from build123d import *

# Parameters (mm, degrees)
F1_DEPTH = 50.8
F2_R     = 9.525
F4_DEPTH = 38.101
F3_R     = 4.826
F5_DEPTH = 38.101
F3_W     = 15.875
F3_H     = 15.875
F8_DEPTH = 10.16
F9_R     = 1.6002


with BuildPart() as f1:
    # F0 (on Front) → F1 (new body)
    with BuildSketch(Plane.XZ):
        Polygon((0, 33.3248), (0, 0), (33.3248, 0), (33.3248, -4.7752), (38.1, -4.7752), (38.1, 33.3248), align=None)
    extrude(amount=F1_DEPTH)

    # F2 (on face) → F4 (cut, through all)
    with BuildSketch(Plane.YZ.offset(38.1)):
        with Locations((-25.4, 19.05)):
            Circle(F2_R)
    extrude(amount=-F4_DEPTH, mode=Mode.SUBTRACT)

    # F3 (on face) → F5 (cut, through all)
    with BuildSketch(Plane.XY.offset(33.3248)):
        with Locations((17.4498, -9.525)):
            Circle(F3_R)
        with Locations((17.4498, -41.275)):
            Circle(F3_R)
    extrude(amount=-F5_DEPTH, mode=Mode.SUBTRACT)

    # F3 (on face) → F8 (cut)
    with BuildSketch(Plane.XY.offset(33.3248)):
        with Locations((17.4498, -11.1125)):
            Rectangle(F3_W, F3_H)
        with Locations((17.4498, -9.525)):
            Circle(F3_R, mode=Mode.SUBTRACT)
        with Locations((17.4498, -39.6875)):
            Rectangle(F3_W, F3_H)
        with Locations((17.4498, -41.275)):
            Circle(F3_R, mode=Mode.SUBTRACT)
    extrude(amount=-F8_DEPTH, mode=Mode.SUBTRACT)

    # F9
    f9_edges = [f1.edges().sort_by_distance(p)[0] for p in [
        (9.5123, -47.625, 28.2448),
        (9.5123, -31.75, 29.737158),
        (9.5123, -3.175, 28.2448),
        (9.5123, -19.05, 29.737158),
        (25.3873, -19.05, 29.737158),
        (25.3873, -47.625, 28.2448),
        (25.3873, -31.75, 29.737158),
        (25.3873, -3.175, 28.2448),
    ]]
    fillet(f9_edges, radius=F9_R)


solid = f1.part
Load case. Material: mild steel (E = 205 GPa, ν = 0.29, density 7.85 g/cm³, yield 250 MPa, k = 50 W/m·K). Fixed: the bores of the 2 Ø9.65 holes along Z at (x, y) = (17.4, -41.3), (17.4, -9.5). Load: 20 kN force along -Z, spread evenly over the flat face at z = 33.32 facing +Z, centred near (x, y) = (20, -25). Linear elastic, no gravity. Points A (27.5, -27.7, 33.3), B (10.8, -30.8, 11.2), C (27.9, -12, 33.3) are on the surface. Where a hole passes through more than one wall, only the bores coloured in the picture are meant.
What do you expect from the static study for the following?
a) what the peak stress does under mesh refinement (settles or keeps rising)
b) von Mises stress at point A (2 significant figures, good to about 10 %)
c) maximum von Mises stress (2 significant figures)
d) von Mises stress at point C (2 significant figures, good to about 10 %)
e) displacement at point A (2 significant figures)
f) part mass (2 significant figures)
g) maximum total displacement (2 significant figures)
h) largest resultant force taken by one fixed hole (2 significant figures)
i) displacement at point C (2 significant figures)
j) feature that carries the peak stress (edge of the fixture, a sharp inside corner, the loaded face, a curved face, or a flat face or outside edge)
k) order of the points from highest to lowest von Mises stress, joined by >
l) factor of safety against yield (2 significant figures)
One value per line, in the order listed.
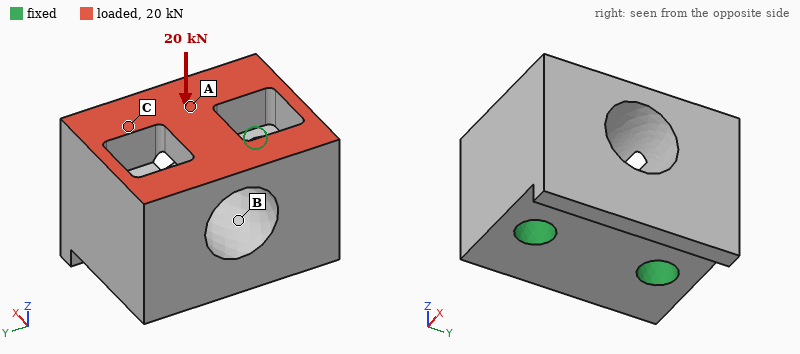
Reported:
settles
64 MPa
280 MPa
35 MPa
9.1 µm
360 g
13 µm
10 kN
4.4 µm
a curved face
A > C > B
0.88
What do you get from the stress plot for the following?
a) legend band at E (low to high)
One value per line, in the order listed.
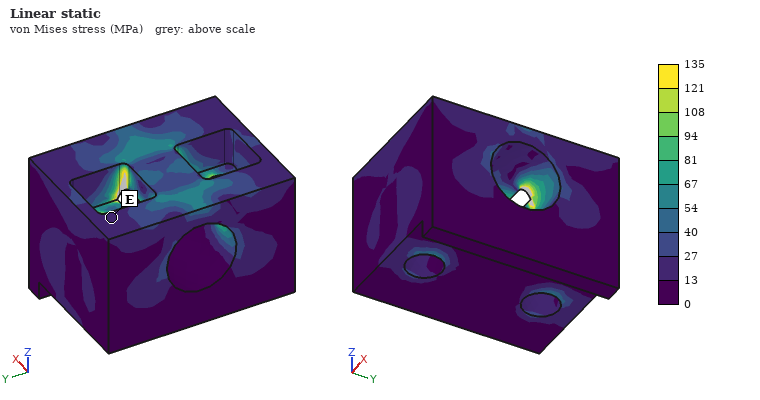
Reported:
13 to 27 MPa
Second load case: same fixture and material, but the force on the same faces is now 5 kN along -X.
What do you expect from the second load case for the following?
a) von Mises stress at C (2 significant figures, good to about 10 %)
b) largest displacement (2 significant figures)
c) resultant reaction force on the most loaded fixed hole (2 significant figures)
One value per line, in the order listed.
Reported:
12 MPa
6.8 µm
2.5 kN
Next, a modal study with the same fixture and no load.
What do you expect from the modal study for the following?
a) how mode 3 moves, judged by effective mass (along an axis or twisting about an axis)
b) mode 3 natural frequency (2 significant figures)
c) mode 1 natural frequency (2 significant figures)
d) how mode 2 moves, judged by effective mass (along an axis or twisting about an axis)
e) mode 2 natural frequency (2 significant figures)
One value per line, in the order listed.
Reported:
twisting about Z
25 kHz
19 kHz
along Y
21 kHz
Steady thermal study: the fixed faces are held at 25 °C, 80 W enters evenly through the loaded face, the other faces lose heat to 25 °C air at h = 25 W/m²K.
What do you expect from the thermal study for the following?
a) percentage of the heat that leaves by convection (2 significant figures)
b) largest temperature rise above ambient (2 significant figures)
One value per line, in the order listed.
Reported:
4.4 %
53 K
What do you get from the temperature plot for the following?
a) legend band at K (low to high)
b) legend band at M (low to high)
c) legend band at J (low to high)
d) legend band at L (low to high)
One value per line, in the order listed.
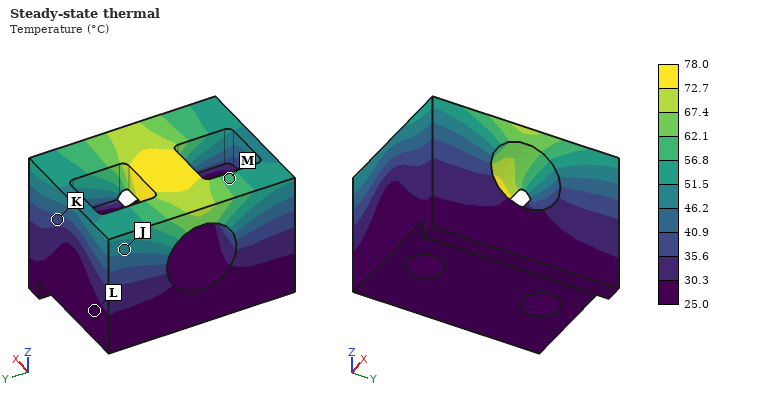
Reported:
35.6 to 40.9 °C
56.8 to 62.1 °C
46.2 to 51.5 °C
25.0 to 30.3 °C
